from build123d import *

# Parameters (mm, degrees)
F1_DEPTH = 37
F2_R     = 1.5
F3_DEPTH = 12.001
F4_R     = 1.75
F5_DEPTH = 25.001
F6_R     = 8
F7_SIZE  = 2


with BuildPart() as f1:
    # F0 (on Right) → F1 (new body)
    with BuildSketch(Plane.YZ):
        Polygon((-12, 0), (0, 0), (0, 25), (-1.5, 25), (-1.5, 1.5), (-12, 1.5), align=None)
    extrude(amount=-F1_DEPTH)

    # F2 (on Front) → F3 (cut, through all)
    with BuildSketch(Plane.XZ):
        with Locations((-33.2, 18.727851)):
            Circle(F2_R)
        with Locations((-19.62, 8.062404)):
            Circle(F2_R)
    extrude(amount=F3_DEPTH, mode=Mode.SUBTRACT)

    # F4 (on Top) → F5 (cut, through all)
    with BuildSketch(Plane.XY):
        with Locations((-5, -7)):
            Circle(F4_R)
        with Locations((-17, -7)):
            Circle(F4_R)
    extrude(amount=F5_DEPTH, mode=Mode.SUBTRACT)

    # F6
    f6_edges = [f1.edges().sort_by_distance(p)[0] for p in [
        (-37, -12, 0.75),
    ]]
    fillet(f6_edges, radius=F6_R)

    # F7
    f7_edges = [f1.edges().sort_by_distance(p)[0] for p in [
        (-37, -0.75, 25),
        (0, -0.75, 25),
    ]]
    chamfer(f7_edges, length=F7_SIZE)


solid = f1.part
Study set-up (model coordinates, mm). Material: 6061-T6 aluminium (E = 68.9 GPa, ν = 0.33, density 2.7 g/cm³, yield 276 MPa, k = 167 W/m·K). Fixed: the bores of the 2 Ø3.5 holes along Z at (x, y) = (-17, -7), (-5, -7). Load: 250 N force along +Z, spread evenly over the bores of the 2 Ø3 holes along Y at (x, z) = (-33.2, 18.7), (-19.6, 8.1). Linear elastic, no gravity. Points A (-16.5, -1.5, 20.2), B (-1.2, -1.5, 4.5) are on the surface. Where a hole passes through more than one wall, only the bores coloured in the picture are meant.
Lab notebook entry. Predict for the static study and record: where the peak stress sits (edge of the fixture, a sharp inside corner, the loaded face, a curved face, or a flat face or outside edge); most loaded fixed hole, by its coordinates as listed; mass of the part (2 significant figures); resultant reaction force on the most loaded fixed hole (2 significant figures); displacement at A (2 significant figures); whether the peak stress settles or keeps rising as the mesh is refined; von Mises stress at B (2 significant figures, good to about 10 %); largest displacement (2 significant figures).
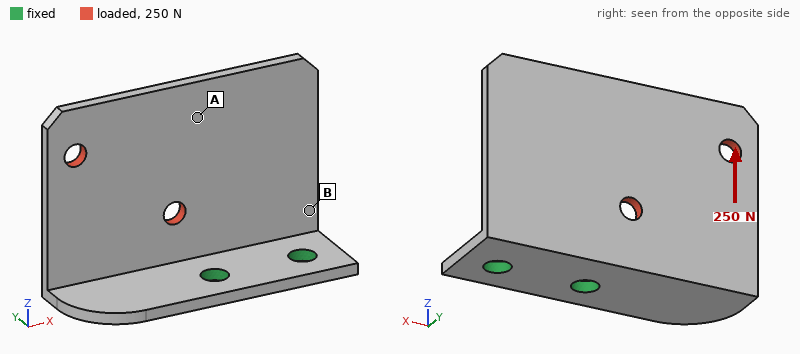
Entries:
edge of the fixture
(-17, -7)
5.1 g
380 N
0.22 mm
keeps rising
77 MPa
0.36 mm
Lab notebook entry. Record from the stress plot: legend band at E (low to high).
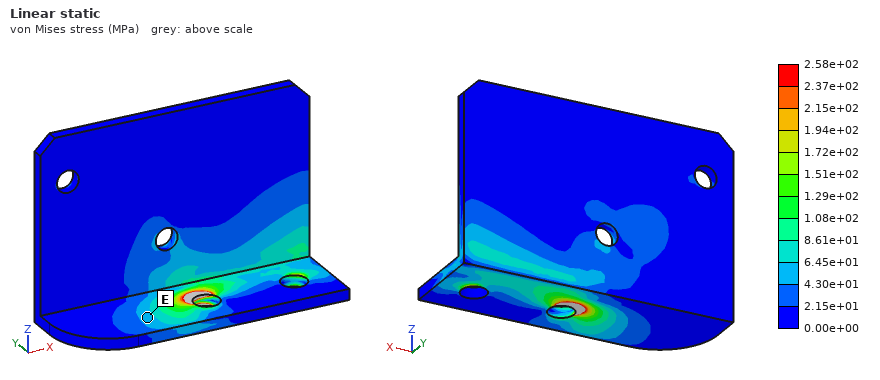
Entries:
4.30e+01 to 6.45e+01 MPa
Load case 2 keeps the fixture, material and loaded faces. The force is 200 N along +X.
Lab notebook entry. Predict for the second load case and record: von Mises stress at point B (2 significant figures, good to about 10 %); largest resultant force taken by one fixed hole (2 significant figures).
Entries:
56 MPa
210 N
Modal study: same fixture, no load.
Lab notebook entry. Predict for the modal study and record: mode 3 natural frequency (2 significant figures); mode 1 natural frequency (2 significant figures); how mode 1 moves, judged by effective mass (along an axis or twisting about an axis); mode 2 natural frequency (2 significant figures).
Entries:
3900 Hz
1500 Hz
along Y
3000 Hz
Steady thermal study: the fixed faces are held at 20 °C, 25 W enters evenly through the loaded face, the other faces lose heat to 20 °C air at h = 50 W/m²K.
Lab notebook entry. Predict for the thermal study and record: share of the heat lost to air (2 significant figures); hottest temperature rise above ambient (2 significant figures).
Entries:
18 %
85 K
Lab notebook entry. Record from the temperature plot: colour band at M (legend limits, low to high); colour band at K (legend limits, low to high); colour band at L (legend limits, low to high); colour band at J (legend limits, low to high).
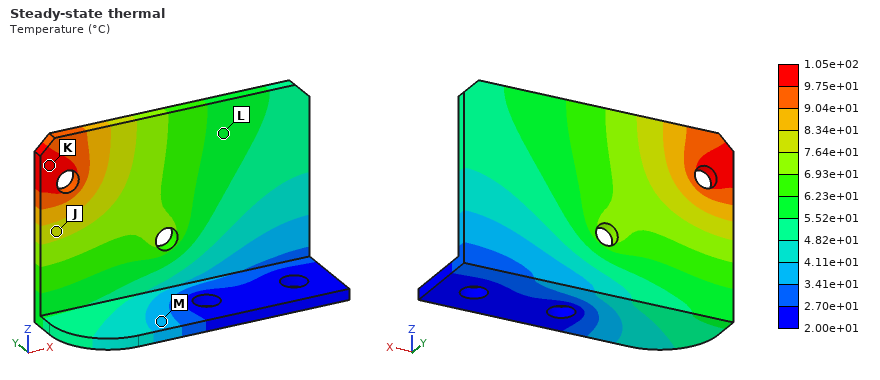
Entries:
3.41e+01 to 4.11e+01 °C
9.75e+01 to 1.05e+02 °C
5.52e+01 to 6.23e+01 °C
7.64e+01 to 8.34e+01 °C
